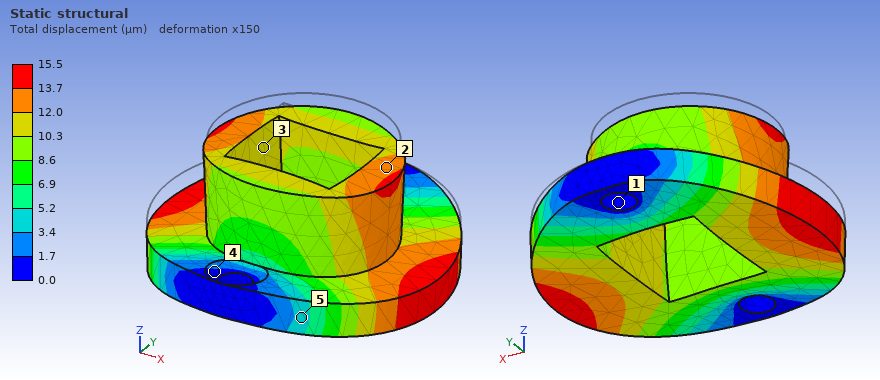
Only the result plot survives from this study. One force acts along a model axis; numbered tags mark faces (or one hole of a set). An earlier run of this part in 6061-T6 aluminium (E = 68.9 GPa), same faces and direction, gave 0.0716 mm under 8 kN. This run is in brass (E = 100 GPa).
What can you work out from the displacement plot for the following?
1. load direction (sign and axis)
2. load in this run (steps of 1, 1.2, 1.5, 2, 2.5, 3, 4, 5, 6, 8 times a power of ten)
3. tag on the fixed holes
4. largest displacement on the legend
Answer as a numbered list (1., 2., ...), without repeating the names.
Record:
1. -Z
2. 2.5 kN
3. 1
4. 15.5 µm
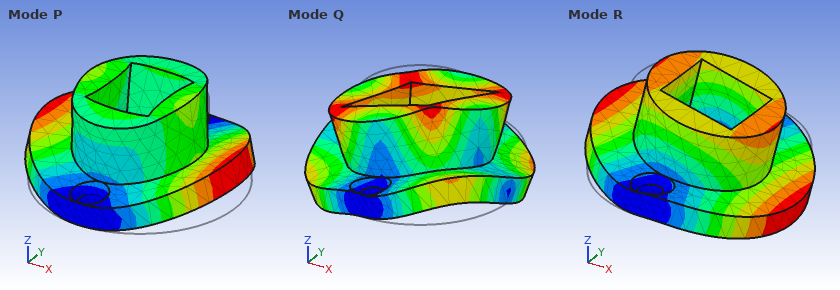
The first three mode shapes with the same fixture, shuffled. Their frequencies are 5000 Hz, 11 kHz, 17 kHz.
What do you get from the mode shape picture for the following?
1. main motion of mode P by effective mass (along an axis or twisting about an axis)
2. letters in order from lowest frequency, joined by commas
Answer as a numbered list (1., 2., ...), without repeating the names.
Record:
1. along Z
2. R, P, Q
